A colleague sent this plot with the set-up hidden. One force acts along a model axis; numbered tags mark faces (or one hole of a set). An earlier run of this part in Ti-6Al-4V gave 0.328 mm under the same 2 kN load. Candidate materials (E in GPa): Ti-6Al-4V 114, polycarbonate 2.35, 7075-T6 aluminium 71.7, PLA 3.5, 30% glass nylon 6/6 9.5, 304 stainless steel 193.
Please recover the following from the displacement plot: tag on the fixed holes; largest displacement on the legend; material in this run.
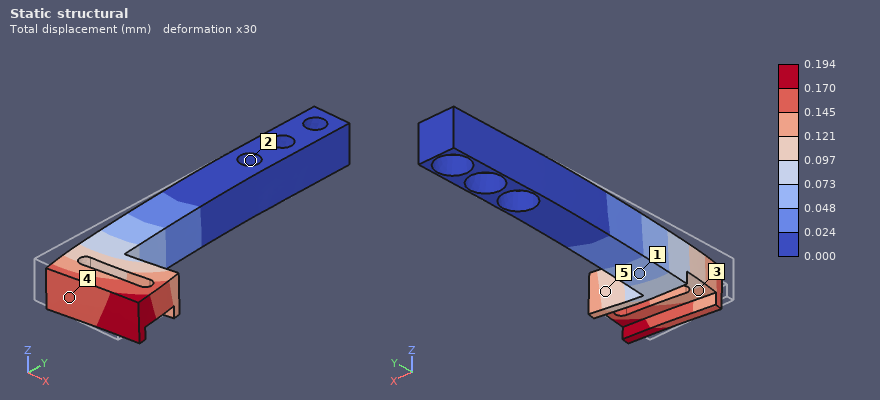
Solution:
2
0.194 mm
304 stainless steel
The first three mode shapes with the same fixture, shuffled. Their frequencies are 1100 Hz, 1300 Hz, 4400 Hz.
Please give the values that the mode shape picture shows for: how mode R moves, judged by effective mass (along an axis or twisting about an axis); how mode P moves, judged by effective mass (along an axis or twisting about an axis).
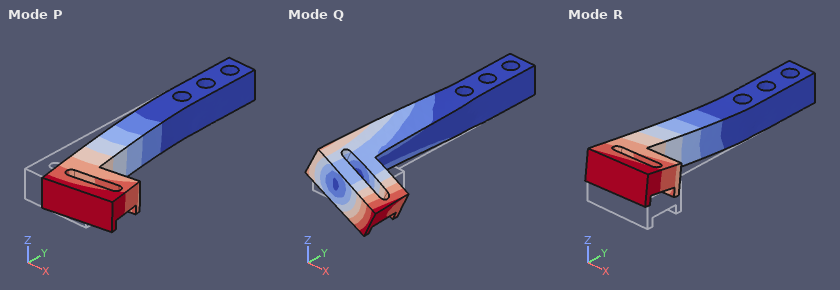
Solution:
along Z
along X
